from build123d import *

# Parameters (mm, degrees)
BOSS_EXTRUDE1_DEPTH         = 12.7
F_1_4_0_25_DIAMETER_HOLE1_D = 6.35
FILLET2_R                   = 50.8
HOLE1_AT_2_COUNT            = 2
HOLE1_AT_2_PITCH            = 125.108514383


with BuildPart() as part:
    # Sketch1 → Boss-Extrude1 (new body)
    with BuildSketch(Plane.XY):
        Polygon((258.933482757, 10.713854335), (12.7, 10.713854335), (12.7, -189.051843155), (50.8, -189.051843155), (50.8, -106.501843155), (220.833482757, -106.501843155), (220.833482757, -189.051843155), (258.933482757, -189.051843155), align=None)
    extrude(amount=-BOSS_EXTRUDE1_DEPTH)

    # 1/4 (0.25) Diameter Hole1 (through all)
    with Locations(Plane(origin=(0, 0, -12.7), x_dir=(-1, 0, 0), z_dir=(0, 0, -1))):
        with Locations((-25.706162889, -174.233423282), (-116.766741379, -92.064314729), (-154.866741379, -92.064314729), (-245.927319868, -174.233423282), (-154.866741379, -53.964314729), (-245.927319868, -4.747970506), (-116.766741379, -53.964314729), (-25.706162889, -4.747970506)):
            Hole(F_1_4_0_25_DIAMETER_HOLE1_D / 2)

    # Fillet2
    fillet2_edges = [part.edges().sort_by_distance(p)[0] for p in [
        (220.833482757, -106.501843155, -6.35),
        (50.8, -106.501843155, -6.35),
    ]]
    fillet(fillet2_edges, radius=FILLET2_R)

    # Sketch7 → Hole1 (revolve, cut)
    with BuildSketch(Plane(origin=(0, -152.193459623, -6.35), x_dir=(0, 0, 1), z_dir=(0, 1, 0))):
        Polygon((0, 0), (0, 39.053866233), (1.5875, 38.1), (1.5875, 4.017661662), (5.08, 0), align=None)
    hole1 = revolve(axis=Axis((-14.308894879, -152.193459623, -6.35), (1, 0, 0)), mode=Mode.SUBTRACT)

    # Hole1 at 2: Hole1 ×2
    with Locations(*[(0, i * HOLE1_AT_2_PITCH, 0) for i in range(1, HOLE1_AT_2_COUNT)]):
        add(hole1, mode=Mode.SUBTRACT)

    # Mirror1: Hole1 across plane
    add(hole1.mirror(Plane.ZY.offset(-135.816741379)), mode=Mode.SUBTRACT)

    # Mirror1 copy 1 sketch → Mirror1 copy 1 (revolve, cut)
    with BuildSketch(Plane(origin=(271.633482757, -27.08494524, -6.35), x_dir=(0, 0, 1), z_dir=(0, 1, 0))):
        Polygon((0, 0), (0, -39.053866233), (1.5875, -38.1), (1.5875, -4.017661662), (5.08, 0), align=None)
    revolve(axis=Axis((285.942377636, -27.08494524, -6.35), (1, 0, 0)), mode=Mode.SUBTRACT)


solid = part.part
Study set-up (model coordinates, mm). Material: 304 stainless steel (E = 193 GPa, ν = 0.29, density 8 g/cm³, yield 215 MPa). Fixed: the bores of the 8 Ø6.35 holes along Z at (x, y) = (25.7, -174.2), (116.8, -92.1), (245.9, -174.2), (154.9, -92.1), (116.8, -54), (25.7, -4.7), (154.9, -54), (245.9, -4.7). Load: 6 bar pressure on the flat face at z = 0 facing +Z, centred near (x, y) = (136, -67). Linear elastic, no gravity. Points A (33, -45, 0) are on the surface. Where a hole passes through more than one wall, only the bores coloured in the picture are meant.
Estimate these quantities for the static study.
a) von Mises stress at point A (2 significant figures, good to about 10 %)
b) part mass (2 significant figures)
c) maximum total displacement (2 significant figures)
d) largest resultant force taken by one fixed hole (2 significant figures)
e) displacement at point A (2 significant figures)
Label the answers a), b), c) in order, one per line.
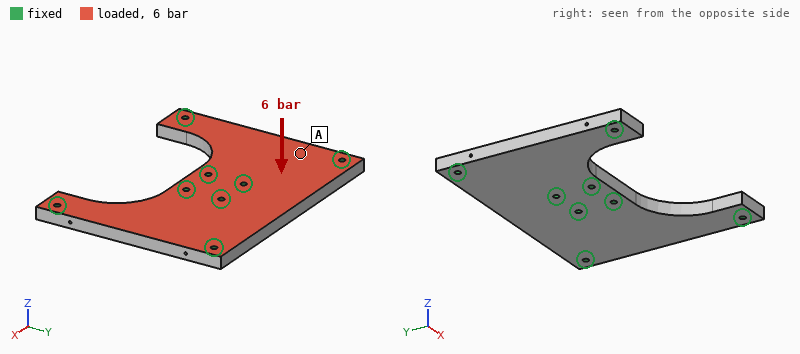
a) 17 MPa
b) 3.7 kg
c) 42 µm
d) 3.6 kN
e) 21 µm
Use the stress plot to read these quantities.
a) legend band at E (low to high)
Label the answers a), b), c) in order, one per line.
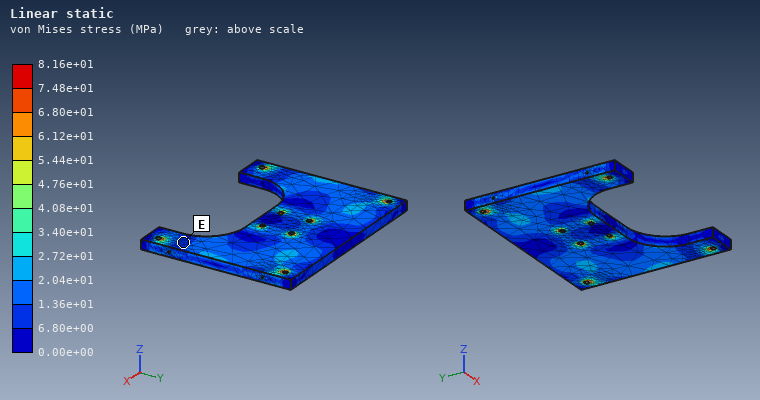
a) 6.80e+00 to 1.36e+01 MPa
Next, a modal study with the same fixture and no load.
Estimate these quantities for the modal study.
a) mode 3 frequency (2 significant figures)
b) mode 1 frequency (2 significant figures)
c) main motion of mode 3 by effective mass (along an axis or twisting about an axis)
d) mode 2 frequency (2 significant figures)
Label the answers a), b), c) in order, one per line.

a) 2900 Hz
b) 2300 Hz
c) along Z
d) 2400 Hz
